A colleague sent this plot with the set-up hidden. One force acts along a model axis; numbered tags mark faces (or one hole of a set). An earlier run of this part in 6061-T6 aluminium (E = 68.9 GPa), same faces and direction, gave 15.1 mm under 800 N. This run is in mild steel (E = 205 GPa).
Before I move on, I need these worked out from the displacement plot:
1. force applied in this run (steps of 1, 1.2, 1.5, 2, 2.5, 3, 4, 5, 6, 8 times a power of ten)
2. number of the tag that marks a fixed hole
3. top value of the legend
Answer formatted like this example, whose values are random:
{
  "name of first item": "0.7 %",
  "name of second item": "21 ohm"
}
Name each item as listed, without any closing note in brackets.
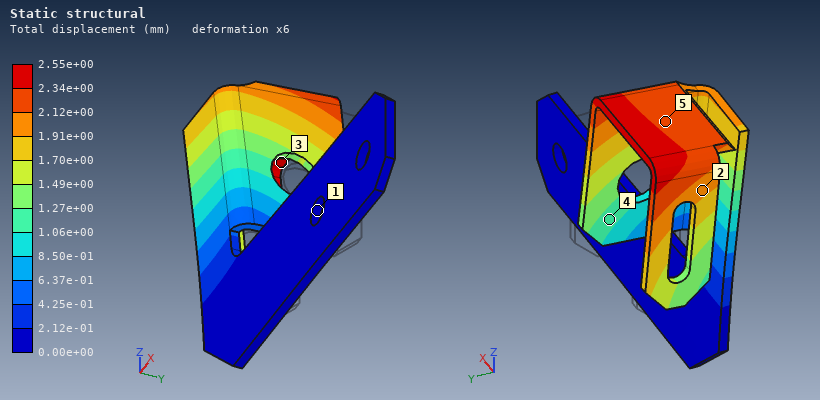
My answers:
{
  "force applied in this run": "400 N",
  "number of the tag that marks a fixed hole": "1",
  "top value of the legend": "2.55e+00 mm"
}
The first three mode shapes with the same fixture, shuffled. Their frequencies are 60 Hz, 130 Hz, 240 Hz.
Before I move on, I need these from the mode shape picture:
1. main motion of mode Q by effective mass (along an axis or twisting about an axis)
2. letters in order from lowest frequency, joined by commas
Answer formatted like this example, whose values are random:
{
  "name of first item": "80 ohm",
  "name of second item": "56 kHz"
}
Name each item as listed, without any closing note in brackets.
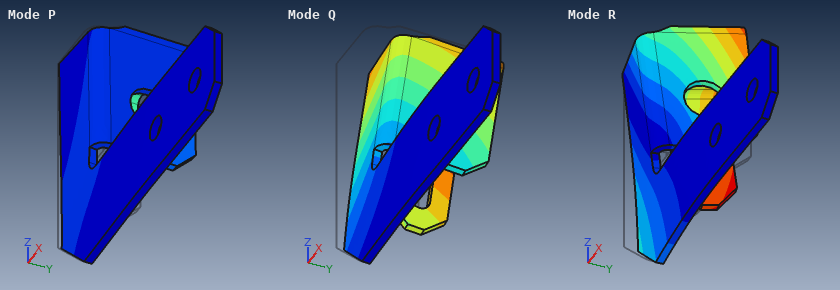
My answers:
{
  "main motion of mode Q by effective mass": "along Y",
  "letters in order from lowest frequency, joined by commas": "Q, R, P"
}
